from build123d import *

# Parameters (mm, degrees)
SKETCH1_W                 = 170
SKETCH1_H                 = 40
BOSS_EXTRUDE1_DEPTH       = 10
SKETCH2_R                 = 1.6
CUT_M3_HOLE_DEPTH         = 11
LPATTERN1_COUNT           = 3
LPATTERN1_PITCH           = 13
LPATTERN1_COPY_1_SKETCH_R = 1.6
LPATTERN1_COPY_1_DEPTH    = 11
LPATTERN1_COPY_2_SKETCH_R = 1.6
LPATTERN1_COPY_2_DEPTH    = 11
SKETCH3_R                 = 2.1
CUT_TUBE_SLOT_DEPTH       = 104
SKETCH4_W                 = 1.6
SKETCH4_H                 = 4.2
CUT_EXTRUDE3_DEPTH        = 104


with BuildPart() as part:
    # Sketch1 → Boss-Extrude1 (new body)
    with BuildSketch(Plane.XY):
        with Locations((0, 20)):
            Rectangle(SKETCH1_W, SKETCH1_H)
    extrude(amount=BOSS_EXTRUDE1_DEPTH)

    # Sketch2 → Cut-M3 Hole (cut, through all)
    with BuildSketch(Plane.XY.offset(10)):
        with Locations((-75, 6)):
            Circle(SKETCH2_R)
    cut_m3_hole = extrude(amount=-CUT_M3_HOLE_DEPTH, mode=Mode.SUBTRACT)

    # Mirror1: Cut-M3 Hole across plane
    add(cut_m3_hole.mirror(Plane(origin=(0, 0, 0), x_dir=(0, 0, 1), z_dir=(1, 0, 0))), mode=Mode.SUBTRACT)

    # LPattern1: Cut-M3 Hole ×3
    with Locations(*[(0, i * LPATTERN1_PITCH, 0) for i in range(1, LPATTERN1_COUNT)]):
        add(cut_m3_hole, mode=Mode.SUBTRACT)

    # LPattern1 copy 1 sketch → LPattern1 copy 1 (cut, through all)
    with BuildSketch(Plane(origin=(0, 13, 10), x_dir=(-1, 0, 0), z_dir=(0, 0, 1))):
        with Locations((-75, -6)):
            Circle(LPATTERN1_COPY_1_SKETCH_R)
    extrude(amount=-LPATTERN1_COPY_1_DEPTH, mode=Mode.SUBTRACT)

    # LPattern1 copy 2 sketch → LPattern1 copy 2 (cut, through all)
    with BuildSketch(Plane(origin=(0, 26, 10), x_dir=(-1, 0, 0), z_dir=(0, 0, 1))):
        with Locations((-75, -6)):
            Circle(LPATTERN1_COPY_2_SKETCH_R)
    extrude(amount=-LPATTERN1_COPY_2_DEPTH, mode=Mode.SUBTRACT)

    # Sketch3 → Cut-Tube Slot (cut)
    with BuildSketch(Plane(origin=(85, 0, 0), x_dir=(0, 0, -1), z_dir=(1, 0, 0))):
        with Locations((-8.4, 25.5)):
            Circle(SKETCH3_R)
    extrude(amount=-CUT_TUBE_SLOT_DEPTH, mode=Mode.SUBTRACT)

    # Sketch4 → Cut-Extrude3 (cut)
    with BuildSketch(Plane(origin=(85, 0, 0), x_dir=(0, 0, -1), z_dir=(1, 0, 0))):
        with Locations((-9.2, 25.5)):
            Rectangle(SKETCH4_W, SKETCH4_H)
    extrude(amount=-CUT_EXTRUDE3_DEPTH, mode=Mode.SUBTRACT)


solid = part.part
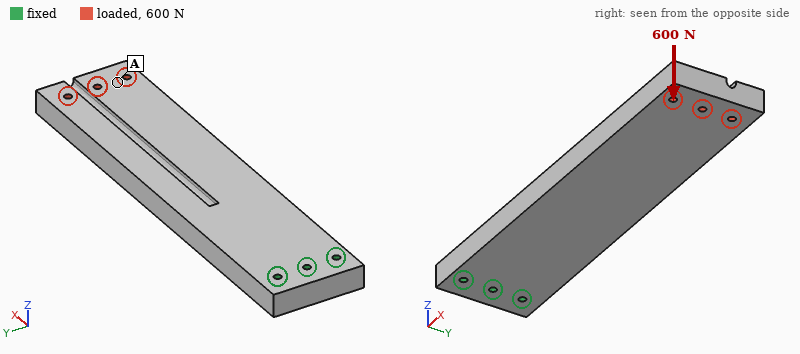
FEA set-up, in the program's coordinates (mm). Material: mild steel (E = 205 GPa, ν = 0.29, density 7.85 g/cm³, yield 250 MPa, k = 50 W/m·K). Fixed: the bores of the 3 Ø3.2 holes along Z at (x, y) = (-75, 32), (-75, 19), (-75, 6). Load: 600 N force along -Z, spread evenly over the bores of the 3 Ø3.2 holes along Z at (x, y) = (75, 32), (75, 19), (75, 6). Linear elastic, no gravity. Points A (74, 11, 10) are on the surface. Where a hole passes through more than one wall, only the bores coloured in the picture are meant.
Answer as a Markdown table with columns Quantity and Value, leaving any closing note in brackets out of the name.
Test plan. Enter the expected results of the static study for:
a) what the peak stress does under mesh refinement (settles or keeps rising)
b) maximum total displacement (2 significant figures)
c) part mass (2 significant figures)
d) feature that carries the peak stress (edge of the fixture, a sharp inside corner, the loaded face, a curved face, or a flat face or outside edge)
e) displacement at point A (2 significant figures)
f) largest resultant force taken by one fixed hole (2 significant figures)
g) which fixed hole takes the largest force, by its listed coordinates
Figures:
| Quantity | Value |
|---|---|
| what the peak stress does under mesh refinement | keeps rising |
| maximum total displacement | 1.1 mm |
| part mass | 520 g |
| feature that carries the peak stress | edge of the fixture |
| displacement at point A | 1.0 mm |
| largest resultant force taken by one fixed hole | 850 N |
| which fixed hole takes the largest force, by its listed coordinates | (-75, 19) |
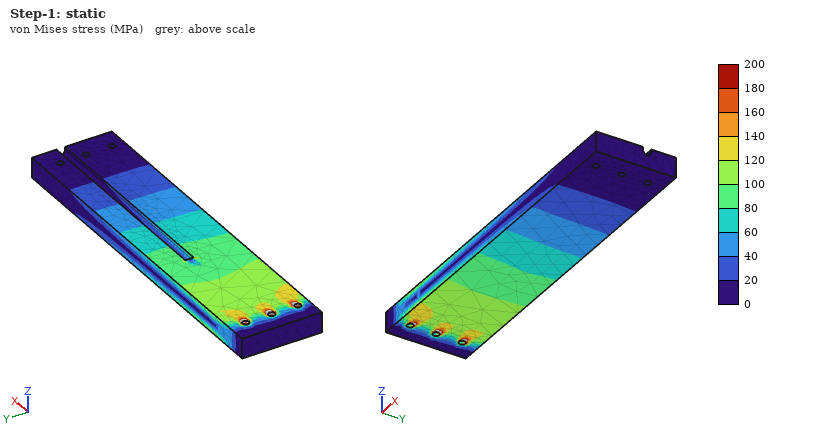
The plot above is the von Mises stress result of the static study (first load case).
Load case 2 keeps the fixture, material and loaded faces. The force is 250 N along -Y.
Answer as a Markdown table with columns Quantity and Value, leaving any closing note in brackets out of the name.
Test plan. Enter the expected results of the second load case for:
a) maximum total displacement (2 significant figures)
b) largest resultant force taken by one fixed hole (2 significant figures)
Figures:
| Quantity | Value |
|---|---|
| maximum total displacement | 32 µm |
| largest resultant force taken by one fixed hole | 1.4 kN |
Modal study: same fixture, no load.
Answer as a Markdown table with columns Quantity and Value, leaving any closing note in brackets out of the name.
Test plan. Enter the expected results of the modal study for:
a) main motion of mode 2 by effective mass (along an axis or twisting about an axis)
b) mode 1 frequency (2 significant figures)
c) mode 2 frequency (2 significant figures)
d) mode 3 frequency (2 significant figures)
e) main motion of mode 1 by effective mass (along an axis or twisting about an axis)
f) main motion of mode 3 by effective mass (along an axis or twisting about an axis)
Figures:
| Quantity | Value |
|---|---|
| main motion of mode 2 by effective mass | along Y |
| mode 1 frequency | 330 Hz |
| mode 2 frequency | 1200 Hz |
| mode 3 frequency | 2000 Hz |
| main motion of mode 1 by effective mass | along Z |
| main motion of mode 3 by effective mass | along Z |
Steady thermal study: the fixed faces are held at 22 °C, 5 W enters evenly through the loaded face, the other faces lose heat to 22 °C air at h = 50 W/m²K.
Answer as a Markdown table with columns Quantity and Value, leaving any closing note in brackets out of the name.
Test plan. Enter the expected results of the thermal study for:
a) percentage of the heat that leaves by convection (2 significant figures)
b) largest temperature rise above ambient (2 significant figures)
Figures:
| Quantity | Value |
|---|---|
| percentage of the heat that leaves by convection | 86 % |
| largest temperature rise above ambient | 13 K |
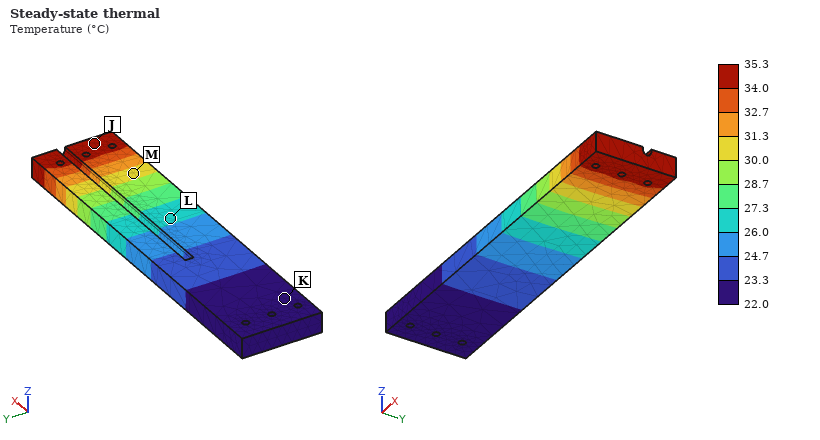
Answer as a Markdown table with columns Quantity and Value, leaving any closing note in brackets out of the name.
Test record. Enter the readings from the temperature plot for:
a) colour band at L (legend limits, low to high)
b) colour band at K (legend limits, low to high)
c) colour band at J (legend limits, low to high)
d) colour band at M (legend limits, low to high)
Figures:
| Quantity | Value |
|---|---|
| colour band at L | 26.0 to 27.3 °C |
| colour band at K | 22.0 to 23.3 °C |
| colour band at J | 34.0 to 35.3 °C |
| colour band at M | 30.0 to 31.3 °C |
